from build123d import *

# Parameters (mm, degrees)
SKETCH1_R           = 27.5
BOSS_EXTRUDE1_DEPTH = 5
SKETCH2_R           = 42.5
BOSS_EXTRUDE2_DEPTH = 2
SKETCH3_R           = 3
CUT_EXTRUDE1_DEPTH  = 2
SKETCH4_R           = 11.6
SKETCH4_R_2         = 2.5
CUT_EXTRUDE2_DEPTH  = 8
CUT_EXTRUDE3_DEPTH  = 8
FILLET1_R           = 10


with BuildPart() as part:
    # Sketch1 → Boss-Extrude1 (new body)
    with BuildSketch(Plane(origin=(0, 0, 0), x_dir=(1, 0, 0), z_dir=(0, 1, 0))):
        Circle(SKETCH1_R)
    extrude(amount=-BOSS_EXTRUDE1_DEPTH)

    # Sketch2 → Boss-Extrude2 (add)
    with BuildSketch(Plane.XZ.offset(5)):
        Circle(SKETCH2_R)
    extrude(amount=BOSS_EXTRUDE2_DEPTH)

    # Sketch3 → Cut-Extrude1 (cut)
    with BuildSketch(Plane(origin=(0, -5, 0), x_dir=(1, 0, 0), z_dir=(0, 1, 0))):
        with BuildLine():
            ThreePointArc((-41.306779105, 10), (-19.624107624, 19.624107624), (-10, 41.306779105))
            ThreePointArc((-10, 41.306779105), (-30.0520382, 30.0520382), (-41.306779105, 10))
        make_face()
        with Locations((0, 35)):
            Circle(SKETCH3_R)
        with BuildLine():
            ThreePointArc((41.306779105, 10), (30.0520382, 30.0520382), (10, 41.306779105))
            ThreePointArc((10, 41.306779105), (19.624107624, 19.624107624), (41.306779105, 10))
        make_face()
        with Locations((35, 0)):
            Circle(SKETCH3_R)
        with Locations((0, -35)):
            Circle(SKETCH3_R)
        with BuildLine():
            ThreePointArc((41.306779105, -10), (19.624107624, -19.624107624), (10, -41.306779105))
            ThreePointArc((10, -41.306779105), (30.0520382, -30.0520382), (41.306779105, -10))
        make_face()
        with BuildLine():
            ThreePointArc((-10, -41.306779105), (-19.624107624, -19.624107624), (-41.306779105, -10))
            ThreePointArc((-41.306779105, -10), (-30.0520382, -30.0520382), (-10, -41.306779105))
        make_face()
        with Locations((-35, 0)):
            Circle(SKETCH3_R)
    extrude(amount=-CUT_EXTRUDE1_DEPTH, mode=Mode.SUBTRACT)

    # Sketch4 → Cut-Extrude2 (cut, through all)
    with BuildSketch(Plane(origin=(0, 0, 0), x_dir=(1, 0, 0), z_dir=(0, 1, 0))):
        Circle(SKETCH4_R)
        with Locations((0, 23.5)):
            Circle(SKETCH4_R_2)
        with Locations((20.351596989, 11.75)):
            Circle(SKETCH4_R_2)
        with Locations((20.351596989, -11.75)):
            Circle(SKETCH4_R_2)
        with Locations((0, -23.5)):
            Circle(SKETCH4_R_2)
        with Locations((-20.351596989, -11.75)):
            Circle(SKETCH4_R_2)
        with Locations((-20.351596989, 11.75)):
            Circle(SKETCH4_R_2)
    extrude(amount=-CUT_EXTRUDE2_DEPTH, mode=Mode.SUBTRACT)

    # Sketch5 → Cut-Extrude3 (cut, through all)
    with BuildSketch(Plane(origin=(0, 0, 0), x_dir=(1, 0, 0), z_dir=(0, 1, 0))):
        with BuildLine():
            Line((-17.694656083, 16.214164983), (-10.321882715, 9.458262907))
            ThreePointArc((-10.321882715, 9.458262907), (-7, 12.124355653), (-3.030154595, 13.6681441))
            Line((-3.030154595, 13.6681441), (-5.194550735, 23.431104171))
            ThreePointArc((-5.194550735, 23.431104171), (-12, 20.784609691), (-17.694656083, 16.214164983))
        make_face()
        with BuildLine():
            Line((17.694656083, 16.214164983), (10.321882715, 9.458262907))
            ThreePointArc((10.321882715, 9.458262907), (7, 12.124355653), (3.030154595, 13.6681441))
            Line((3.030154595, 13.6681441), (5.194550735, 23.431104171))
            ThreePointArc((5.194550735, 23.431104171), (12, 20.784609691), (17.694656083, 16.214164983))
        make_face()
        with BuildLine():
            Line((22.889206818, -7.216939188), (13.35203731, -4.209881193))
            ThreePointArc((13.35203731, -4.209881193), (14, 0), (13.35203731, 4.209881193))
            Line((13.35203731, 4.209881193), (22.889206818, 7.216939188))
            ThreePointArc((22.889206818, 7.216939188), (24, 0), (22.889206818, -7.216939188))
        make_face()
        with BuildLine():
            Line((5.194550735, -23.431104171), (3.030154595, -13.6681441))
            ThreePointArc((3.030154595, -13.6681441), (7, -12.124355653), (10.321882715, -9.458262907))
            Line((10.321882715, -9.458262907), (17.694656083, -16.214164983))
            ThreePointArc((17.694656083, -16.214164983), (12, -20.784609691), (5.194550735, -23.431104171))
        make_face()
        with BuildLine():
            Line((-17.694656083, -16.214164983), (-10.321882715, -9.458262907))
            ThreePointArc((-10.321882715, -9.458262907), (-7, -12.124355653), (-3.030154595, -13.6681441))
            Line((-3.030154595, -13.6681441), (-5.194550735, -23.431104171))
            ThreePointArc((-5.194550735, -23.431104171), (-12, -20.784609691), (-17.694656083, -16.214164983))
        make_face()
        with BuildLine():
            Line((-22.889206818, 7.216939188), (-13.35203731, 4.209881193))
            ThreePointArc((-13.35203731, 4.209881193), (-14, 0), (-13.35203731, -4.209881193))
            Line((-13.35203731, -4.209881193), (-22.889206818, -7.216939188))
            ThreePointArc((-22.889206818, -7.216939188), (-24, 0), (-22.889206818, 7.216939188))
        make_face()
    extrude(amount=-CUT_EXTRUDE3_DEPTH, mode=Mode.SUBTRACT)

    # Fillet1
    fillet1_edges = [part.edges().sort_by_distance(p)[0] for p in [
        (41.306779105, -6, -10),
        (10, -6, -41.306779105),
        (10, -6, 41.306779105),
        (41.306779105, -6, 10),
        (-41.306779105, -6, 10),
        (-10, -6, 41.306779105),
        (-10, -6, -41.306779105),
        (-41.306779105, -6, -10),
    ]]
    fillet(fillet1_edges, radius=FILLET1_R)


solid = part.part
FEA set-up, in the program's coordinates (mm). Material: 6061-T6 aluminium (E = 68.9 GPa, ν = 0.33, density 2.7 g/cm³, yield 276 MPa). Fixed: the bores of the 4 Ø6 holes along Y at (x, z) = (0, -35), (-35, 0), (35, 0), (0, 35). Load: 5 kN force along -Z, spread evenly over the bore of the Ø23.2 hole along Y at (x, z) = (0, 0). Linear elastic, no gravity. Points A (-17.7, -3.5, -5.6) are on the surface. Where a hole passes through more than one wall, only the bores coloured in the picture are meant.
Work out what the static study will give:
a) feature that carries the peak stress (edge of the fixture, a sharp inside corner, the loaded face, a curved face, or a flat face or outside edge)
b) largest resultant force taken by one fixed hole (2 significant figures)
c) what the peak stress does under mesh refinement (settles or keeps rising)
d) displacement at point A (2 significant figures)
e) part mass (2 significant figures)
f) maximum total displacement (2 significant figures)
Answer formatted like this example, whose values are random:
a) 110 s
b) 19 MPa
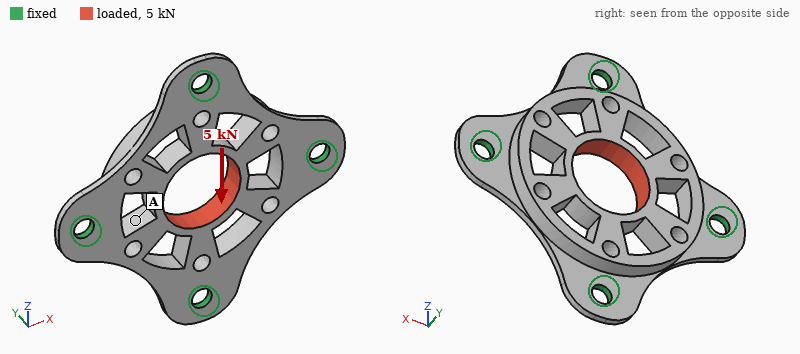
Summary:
a) edge of the fixture
b) 1.6 kN
c) keeps rising
d) 30 µm
e) 29 g
f) 46 µm
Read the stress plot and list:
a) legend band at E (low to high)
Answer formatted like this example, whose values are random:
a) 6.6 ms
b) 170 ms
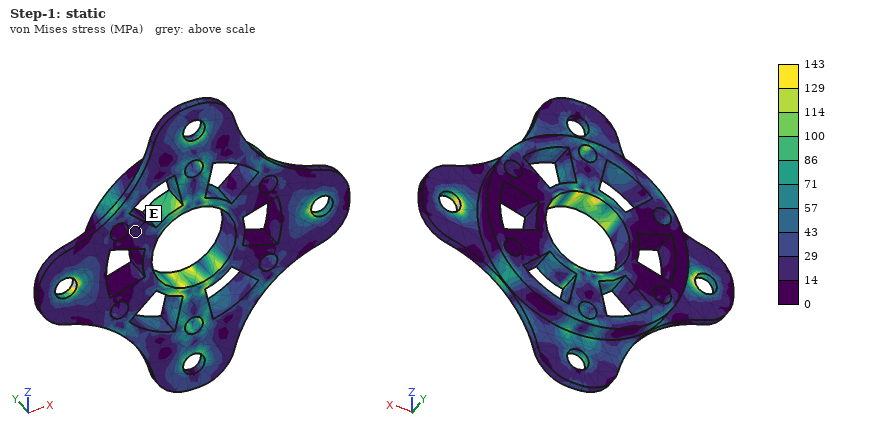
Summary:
a) 14 to 29 MPa
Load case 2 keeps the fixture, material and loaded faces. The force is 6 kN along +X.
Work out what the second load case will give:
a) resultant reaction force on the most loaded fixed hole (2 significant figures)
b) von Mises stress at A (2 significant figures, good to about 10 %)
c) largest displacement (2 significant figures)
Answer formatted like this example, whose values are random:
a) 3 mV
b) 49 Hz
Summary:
a) 2.1 kN
b) 60 MPa
c) 42 µm
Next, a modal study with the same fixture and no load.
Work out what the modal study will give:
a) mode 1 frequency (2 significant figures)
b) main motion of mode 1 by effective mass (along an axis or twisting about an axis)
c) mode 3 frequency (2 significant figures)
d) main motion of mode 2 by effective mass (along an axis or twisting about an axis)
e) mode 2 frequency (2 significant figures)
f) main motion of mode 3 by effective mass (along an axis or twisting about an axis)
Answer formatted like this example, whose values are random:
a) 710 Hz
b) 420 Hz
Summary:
a) 6200 Hz
b) along Y
c) 8900 Hz
d) twisting about X
e) 8500 Hz
f) twisting about Z
